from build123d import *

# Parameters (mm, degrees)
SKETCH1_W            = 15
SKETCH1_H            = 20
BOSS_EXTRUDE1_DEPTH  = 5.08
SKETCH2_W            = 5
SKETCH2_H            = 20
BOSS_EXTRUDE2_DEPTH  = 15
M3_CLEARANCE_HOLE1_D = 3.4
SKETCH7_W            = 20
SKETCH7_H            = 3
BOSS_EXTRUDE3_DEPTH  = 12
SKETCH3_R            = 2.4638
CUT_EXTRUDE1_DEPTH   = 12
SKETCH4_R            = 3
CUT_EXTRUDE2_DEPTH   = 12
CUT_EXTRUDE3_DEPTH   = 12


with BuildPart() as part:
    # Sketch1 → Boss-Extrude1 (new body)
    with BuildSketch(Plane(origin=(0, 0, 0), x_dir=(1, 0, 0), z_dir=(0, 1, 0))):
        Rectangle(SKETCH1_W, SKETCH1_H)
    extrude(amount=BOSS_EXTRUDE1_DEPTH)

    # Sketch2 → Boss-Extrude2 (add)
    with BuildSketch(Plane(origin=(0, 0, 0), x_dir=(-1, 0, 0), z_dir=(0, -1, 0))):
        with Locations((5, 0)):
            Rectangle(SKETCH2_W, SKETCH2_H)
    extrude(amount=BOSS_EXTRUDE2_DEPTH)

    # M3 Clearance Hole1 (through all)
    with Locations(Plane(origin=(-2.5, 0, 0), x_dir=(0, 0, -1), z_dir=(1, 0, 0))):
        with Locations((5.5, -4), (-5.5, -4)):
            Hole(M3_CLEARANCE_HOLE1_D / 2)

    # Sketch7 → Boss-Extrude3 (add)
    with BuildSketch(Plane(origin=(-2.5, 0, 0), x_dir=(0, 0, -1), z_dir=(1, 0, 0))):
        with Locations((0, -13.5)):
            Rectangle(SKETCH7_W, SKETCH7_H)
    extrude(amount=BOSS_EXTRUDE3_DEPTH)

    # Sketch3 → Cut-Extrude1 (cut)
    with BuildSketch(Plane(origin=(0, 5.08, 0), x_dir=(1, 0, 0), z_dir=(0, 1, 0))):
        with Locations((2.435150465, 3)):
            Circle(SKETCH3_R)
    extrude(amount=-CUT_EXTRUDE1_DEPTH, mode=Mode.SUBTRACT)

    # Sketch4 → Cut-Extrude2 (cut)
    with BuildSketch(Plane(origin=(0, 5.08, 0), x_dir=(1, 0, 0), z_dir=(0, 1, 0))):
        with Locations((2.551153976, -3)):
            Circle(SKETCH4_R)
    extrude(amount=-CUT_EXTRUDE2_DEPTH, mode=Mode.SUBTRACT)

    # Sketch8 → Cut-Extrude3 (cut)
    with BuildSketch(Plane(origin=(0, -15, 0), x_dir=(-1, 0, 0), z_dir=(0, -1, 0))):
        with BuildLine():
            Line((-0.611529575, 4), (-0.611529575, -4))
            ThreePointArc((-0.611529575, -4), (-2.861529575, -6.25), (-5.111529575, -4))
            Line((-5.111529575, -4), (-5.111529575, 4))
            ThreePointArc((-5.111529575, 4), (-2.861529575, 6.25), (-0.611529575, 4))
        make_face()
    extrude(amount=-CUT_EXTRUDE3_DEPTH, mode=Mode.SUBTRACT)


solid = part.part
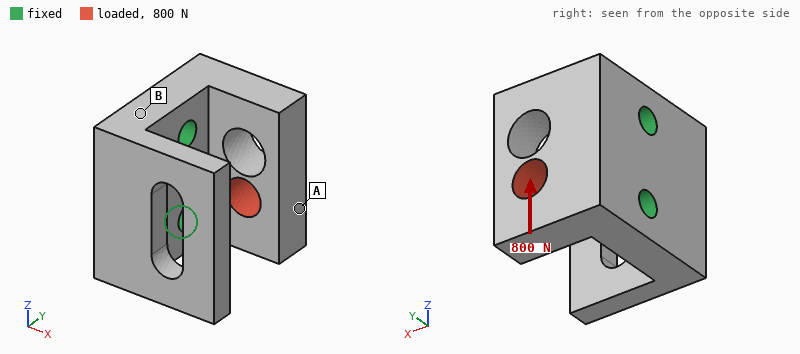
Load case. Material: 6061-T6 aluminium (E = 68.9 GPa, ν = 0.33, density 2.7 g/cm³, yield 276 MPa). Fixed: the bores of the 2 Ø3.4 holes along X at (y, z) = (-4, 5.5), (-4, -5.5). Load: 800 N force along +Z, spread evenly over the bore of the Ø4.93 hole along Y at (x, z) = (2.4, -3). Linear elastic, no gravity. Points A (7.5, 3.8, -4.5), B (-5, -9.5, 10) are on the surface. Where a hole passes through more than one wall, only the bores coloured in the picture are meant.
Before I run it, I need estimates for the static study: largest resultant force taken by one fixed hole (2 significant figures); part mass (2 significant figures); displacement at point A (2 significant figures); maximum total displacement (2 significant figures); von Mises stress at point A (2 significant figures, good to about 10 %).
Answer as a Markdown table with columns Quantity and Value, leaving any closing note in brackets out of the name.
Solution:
| Quantity | Value |
|---|---|
| largest resultant force taken by one fixed hole | 660 N |
| part mass | 8.8 g |
| displacement at point A | 19 µm |
| maximum total displacement | 22 µm |
| von Mises stress at point A | 32 MPa |
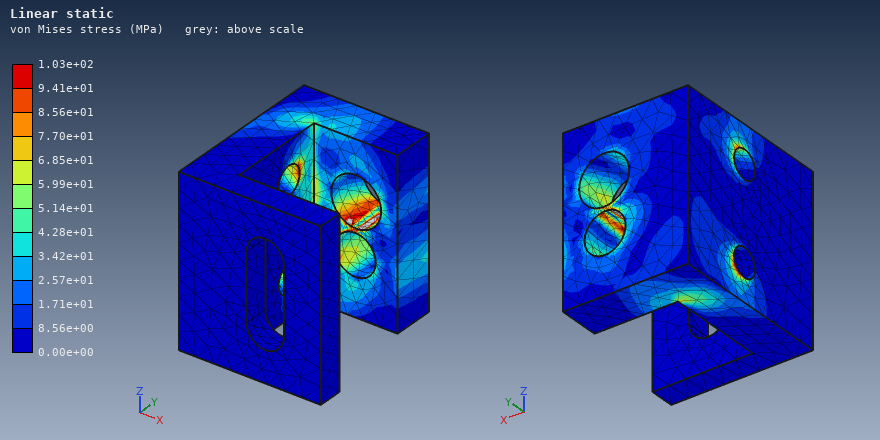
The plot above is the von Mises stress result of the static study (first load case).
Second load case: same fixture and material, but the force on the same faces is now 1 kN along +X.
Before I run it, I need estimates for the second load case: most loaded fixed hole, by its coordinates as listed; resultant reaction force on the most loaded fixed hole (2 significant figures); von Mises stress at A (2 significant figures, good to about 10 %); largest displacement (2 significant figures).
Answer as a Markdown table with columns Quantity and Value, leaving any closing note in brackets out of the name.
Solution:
| Quantity | Value |
|---|---|
| most loaded fixed hole, by its coordinates as listed | (-4, -5.5) |
| resultant reaction force on the most loaded fixed hole | 710 N |
| von Mises stress at A | 20 MPa |
| largest displacement | 26 µm |
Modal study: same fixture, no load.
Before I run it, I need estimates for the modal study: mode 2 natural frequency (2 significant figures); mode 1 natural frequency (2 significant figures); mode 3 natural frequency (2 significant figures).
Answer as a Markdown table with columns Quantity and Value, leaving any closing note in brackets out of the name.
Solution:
| Quantity | Value |
|---|---|
| mode 2 natural frequency | 16 kHz |
| mode 1 natural frequency | 9000 Hz |
| mode 3 natural frequency | 16 kHz |
